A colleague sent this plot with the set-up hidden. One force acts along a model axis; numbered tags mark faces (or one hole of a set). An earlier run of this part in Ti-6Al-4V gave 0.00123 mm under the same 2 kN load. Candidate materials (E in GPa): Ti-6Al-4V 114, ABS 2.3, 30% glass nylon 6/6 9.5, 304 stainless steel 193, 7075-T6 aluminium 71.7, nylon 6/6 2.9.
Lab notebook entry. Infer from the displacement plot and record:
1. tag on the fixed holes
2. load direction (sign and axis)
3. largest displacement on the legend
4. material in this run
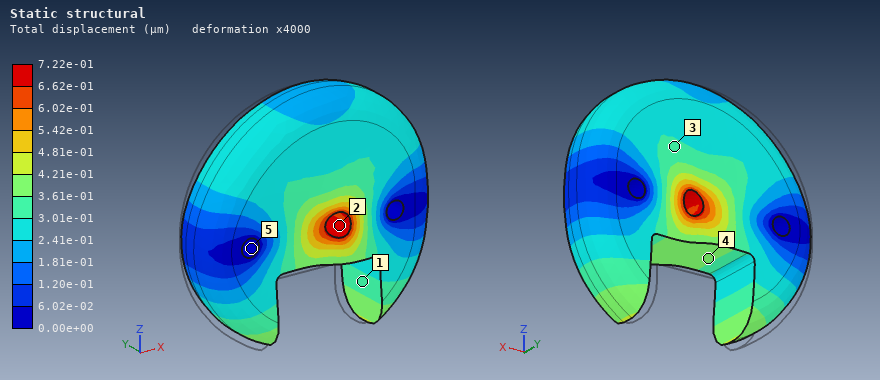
5
+X
7.22e-01 µm
304 stainless steel
